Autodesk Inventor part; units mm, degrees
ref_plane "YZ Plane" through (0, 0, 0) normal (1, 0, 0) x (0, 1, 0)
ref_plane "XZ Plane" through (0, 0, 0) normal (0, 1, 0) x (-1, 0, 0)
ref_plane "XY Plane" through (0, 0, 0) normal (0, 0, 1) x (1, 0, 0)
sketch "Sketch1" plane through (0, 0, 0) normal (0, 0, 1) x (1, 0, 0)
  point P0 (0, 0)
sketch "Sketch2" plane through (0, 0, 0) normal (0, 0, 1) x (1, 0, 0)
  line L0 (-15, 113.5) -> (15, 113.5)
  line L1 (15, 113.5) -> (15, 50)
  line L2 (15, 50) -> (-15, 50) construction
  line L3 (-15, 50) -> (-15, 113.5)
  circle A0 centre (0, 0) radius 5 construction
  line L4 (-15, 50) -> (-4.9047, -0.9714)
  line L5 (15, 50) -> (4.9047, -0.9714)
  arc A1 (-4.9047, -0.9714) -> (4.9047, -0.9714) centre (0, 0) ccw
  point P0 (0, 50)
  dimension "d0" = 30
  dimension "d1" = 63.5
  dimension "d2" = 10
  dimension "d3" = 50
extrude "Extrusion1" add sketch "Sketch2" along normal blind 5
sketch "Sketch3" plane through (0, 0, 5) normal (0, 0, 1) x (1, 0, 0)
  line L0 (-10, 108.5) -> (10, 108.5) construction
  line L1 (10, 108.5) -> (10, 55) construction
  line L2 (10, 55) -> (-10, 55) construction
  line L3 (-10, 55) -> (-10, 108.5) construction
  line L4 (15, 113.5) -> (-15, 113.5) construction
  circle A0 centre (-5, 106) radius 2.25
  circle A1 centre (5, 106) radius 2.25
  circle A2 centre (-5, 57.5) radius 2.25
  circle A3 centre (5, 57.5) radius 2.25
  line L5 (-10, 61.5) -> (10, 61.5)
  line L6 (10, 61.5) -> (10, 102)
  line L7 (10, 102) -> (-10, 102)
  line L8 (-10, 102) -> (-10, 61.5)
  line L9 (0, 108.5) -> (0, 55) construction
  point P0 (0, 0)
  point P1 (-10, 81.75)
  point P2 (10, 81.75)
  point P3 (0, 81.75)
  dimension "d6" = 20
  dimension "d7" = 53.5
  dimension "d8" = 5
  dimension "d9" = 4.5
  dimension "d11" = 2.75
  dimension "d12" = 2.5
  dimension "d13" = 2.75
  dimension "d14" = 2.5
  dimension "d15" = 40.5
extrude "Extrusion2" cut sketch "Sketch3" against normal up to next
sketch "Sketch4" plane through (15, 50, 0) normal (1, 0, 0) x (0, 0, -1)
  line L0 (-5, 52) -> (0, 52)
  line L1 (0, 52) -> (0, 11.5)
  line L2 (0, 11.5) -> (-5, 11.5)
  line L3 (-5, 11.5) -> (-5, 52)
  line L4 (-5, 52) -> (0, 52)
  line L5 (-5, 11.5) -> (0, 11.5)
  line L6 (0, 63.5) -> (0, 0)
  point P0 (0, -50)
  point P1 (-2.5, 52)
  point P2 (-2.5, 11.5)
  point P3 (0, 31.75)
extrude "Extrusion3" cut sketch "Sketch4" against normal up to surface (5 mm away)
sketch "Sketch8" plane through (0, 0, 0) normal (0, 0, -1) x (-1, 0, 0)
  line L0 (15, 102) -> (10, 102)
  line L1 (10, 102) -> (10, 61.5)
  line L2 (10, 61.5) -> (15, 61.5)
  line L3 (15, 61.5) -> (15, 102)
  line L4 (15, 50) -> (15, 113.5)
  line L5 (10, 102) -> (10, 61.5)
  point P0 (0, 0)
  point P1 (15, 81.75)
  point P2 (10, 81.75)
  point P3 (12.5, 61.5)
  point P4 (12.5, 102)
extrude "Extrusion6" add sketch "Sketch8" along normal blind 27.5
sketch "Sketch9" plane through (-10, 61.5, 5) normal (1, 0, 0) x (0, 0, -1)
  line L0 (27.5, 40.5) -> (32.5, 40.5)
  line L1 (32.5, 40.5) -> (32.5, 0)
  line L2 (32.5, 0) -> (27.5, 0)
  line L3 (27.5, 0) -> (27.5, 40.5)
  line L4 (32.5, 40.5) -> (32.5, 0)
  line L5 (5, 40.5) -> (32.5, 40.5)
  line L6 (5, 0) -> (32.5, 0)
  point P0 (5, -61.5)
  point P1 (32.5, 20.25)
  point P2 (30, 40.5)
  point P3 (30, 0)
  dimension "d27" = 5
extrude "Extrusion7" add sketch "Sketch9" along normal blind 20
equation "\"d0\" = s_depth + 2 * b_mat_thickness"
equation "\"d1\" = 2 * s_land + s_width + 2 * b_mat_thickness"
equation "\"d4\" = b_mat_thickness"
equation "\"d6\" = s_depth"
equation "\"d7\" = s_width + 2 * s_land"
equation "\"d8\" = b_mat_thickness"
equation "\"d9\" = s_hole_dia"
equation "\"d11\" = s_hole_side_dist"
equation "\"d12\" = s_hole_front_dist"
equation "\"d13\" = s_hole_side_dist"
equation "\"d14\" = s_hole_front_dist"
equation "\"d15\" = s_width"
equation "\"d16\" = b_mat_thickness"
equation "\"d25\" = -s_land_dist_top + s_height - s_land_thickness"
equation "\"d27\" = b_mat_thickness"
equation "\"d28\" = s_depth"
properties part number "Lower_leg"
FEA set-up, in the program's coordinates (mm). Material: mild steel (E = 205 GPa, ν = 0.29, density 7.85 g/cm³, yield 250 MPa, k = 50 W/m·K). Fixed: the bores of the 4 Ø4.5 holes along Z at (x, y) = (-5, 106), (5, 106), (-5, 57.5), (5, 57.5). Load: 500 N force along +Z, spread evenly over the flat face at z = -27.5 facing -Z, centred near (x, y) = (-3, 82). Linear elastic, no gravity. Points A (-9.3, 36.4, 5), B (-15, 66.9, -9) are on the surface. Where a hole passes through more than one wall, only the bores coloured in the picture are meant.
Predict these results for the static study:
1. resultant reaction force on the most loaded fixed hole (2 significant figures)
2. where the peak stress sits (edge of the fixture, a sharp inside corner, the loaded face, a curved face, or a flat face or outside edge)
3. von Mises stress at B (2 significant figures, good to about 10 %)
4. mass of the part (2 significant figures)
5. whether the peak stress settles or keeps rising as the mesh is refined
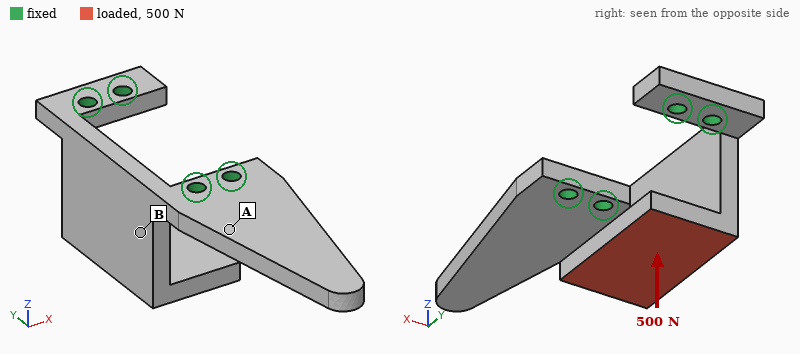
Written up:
260 N
a sharp inside corner
29 MPa
150 g
keeps rising
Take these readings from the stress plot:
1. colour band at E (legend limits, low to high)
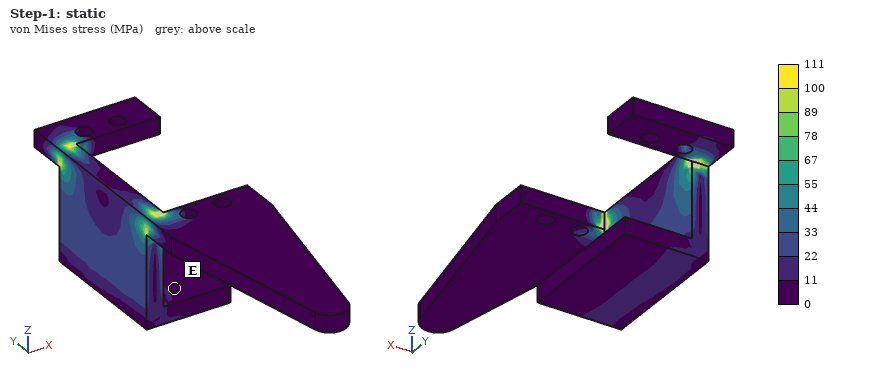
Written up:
0 to 11 MPa
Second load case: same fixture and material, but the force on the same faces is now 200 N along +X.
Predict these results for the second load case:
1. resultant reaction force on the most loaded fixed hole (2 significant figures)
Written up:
120 N
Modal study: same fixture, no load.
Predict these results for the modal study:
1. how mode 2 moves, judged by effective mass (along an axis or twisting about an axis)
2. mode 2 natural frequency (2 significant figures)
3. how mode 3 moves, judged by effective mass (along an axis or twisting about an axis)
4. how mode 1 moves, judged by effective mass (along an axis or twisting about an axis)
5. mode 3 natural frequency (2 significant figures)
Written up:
along Z
1600 Hz
along Y
along X
3300 Hz
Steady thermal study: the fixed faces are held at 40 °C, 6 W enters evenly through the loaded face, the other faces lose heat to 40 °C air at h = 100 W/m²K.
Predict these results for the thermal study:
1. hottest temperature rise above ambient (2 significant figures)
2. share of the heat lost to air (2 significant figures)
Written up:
16 K
74 %
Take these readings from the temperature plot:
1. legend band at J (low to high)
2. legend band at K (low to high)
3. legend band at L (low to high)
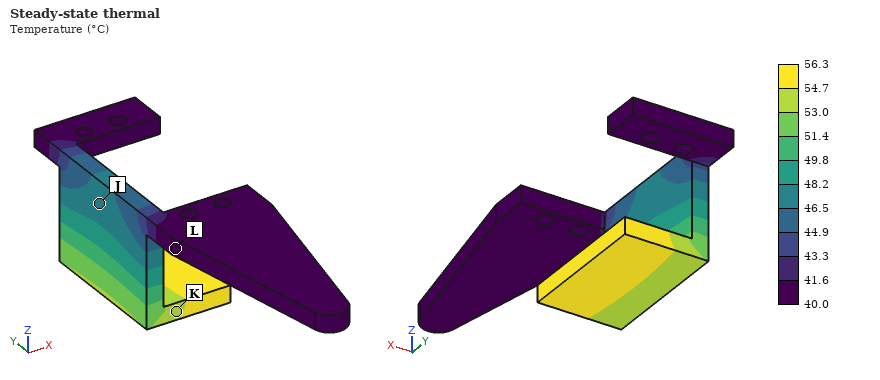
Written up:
46.5 to 48.2 °C
53.0 to 54.7 °C
40.0 to 41.6 °C
